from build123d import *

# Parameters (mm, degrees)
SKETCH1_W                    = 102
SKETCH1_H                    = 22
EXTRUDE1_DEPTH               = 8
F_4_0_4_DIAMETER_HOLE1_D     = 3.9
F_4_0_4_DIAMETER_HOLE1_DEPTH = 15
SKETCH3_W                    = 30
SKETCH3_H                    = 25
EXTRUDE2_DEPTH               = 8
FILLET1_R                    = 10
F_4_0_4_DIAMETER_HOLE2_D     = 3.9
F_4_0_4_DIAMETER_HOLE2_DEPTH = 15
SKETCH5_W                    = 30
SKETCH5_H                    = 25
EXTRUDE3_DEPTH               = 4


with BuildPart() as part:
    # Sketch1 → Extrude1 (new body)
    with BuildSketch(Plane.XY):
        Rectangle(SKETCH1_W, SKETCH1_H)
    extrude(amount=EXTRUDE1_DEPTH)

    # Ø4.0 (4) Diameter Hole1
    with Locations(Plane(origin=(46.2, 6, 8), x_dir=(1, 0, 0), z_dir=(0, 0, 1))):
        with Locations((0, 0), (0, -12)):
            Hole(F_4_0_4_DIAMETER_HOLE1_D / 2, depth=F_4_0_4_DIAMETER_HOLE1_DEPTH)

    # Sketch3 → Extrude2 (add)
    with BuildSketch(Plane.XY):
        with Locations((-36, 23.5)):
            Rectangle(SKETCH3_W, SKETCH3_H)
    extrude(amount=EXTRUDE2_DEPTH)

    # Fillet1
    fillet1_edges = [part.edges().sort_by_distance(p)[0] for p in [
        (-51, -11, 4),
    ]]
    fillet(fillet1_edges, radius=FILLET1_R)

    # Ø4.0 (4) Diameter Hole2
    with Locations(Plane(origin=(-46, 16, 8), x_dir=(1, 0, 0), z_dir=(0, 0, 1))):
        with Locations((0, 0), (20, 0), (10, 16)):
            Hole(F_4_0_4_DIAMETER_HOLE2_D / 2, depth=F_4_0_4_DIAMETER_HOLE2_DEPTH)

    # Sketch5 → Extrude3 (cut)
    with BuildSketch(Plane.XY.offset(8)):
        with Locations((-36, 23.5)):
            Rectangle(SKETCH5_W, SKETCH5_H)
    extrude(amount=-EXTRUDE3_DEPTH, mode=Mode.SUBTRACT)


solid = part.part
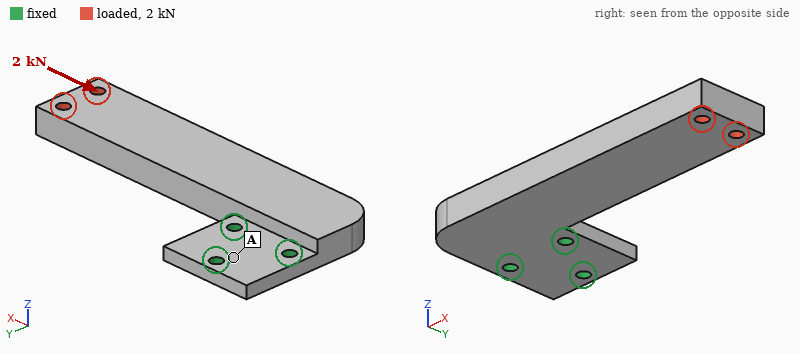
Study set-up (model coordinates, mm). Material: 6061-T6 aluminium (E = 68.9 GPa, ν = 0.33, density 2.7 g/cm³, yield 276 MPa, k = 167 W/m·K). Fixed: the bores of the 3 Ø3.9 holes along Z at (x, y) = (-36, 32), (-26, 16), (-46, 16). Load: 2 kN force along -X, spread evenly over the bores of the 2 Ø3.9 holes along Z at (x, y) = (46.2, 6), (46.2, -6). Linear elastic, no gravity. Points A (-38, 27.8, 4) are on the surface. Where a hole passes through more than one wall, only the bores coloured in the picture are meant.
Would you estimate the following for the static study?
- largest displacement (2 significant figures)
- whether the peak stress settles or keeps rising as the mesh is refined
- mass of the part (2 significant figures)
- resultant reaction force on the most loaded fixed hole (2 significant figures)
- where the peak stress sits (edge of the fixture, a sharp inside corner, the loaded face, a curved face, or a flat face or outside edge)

61 µm
keeps rising
55 g
1.8 kN
edge of the fixture
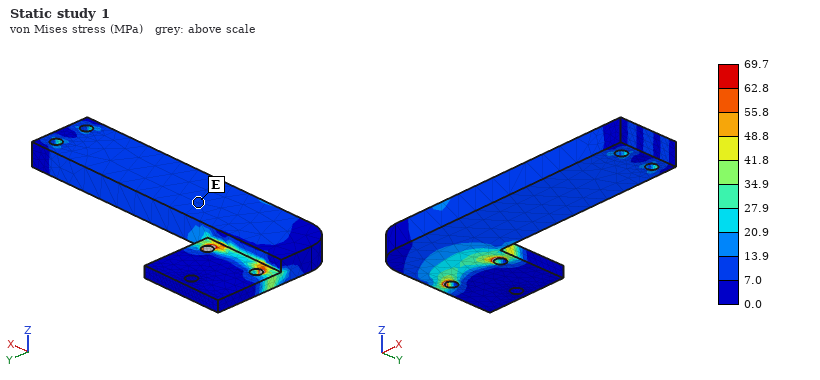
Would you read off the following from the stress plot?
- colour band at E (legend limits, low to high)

7.0 to 13.9 MPa
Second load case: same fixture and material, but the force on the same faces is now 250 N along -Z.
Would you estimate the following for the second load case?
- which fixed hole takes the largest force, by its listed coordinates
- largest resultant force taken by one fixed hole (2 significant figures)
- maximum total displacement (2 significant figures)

(-26, 16)
1.0 kN
0.91 mm
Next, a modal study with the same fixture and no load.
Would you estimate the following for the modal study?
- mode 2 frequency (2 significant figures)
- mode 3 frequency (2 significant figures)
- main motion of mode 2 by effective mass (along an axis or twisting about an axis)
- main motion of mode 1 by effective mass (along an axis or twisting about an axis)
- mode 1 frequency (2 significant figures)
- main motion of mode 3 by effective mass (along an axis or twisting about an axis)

2100 Hz
2700 Hz
along Y
along Z
800 Hz
along Z
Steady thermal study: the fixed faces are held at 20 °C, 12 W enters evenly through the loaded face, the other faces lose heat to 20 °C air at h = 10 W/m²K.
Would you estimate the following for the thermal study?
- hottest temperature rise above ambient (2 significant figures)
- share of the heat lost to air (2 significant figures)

35 K
9.0 %
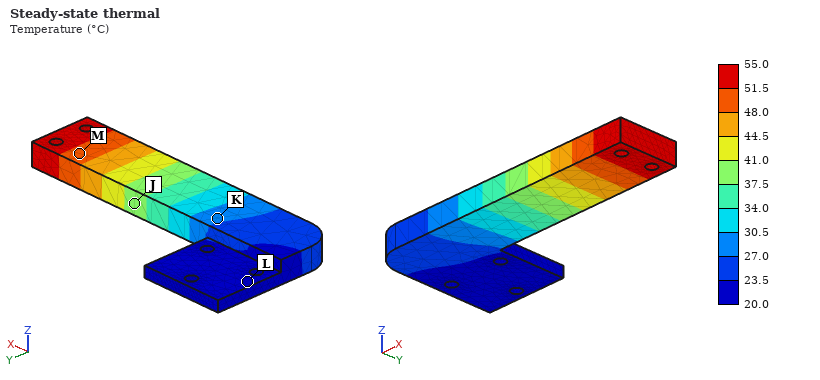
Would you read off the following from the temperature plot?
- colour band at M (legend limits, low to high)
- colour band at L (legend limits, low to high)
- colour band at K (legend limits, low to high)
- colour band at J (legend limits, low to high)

48.0 to 51.5 °C
20.0 to 23.5 °C
27.0 to 30.5 °C
37.5 to 41.0 °C
